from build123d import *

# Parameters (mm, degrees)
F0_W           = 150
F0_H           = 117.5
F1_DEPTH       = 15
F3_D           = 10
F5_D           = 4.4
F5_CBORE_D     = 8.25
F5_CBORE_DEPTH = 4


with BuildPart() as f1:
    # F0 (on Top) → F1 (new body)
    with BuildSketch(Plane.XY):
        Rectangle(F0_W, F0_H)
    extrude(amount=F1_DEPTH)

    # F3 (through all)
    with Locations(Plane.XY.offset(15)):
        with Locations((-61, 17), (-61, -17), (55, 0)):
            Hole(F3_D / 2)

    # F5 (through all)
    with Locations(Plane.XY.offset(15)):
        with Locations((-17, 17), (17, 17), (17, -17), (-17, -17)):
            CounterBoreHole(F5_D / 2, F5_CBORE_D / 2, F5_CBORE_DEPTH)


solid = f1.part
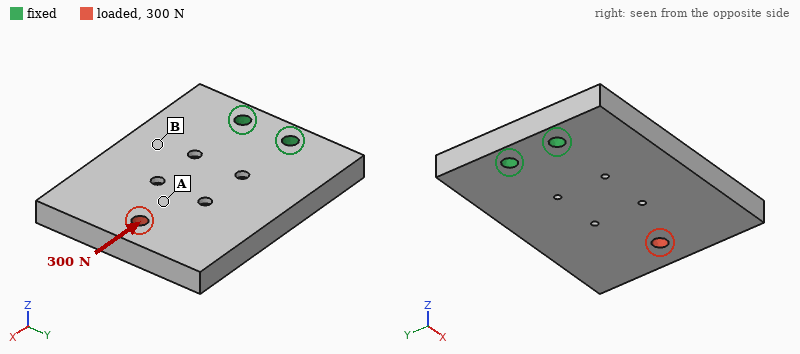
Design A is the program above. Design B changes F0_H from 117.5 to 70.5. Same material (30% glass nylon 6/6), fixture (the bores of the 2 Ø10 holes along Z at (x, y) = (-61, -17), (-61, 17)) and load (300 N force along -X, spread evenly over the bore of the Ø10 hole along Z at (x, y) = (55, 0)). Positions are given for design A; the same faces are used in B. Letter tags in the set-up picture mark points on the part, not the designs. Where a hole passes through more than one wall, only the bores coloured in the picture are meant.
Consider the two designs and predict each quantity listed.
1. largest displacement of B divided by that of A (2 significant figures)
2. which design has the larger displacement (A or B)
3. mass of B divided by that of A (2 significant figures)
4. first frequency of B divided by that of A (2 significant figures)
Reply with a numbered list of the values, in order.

1. 1.1
2. B
3. 0.59
4. 1.1
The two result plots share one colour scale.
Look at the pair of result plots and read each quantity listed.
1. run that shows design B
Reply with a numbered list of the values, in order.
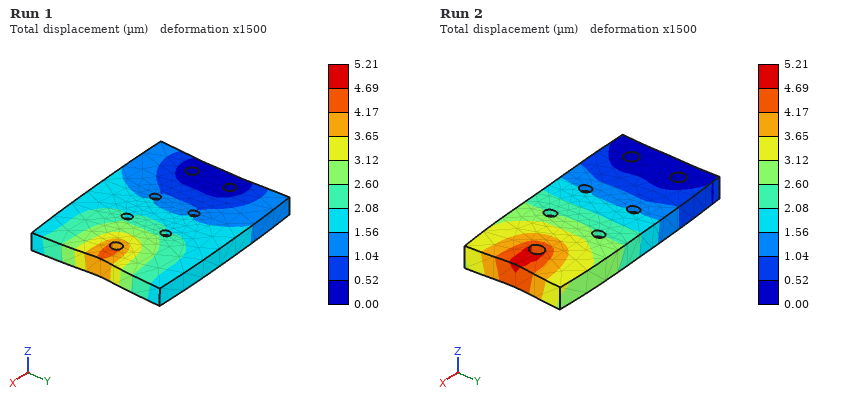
1. Run 2
